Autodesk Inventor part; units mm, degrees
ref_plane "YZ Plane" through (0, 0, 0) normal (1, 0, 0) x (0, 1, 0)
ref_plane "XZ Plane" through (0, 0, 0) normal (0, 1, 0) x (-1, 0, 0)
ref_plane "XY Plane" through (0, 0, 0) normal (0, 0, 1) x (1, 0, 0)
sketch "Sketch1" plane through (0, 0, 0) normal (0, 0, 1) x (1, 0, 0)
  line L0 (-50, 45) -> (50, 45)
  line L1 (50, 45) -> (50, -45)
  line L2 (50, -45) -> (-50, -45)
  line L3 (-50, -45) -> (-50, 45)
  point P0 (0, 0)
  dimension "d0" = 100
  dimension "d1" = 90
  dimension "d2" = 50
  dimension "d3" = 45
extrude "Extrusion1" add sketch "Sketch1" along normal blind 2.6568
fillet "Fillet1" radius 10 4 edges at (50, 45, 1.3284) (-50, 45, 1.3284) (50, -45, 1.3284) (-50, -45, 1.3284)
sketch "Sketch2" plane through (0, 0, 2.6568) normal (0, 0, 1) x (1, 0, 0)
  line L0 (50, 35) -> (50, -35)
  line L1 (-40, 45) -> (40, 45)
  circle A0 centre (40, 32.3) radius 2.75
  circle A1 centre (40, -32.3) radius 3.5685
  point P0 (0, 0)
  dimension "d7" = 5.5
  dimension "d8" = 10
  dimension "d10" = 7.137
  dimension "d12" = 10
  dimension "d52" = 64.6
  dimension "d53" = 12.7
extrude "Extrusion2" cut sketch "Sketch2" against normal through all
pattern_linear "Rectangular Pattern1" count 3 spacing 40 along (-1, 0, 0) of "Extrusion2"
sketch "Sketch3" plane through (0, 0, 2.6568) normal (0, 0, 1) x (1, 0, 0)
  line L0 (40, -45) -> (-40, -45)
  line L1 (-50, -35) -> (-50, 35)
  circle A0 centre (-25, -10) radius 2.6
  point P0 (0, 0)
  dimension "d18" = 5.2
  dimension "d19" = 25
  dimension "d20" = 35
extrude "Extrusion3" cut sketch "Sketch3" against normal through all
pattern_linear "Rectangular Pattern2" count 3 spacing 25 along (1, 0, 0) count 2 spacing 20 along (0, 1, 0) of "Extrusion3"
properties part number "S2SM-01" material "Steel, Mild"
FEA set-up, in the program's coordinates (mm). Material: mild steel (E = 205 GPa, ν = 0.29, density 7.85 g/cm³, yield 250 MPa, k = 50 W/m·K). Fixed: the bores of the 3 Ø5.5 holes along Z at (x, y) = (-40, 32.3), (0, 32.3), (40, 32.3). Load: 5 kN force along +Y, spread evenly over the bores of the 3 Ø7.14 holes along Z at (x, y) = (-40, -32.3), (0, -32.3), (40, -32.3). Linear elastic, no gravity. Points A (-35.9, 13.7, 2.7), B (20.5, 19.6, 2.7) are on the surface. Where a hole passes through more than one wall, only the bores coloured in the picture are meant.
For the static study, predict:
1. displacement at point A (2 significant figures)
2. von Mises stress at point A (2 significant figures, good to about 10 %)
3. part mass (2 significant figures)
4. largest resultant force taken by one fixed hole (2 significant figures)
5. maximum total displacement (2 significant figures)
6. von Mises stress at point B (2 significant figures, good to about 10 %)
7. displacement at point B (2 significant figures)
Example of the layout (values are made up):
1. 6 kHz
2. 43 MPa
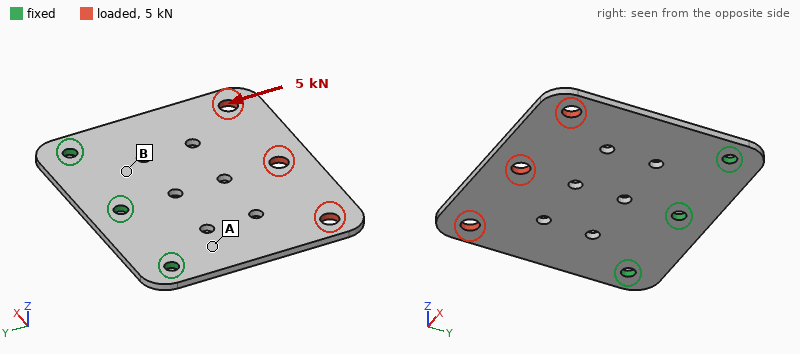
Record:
1. 2.6 µm
2. 23 MPa
3. 180 g
4. 1.8 kN
5. 9.4 µm
6. 11 MPa
7. 2.4 µm
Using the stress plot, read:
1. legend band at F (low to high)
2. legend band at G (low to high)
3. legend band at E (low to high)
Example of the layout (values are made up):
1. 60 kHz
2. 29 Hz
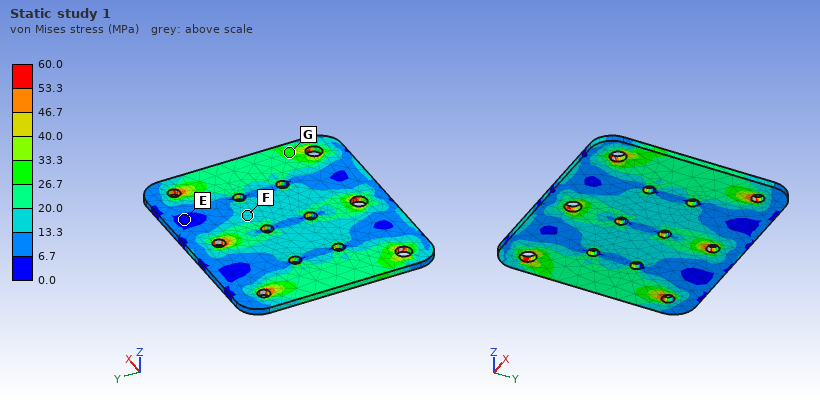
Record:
1. 13.3 to 20.0 MPa
2. 26.7 to 33.3 MPa
3. 0.0 to 6.7 MPa
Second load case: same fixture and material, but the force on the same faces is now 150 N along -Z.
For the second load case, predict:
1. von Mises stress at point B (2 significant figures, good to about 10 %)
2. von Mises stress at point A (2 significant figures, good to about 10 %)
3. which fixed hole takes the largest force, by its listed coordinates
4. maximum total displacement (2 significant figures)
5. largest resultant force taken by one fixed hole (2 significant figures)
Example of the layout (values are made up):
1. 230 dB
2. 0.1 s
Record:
1. 56 MPa
2. 57 MPa
3. (0, 32.3)
4. 0.55 mm
5. 73 N
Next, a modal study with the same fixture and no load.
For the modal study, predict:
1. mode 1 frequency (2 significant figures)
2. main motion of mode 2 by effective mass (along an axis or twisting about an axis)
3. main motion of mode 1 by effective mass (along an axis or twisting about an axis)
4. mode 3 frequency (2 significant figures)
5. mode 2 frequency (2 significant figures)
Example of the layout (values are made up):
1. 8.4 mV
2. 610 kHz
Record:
1. 380 Hz
2. twisting about Y
3. along Z
4. 1900 Hz
5. 790 Hz
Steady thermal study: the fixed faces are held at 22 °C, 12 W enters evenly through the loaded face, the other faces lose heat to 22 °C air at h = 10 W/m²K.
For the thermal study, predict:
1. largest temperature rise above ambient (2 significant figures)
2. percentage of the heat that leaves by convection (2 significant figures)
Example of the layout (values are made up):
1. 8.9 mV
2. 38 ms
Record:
1. 54 K
2. 36 %
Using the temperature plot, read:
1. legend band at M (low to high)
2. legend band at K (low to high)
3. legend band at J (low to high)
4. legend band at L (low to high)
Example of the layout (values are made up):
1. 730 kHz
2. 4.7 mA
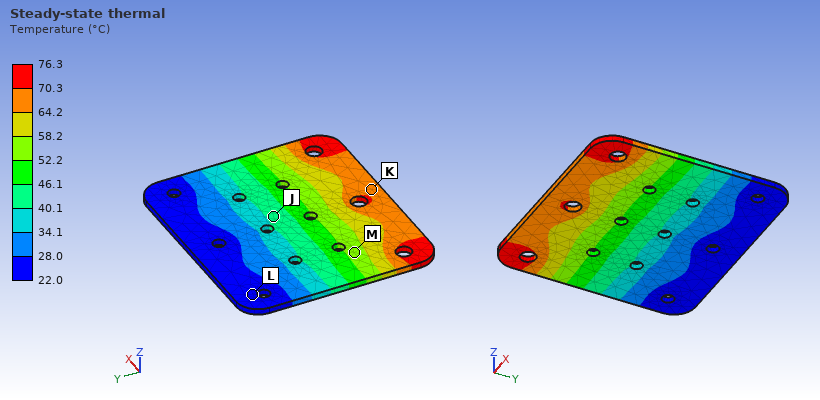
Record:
1. 52.2 to 58.2 °C
2. 64.2 to 70.3 °C
3. 40.1 to 46.1 °C
4. 22.0 to 28.0 °C
